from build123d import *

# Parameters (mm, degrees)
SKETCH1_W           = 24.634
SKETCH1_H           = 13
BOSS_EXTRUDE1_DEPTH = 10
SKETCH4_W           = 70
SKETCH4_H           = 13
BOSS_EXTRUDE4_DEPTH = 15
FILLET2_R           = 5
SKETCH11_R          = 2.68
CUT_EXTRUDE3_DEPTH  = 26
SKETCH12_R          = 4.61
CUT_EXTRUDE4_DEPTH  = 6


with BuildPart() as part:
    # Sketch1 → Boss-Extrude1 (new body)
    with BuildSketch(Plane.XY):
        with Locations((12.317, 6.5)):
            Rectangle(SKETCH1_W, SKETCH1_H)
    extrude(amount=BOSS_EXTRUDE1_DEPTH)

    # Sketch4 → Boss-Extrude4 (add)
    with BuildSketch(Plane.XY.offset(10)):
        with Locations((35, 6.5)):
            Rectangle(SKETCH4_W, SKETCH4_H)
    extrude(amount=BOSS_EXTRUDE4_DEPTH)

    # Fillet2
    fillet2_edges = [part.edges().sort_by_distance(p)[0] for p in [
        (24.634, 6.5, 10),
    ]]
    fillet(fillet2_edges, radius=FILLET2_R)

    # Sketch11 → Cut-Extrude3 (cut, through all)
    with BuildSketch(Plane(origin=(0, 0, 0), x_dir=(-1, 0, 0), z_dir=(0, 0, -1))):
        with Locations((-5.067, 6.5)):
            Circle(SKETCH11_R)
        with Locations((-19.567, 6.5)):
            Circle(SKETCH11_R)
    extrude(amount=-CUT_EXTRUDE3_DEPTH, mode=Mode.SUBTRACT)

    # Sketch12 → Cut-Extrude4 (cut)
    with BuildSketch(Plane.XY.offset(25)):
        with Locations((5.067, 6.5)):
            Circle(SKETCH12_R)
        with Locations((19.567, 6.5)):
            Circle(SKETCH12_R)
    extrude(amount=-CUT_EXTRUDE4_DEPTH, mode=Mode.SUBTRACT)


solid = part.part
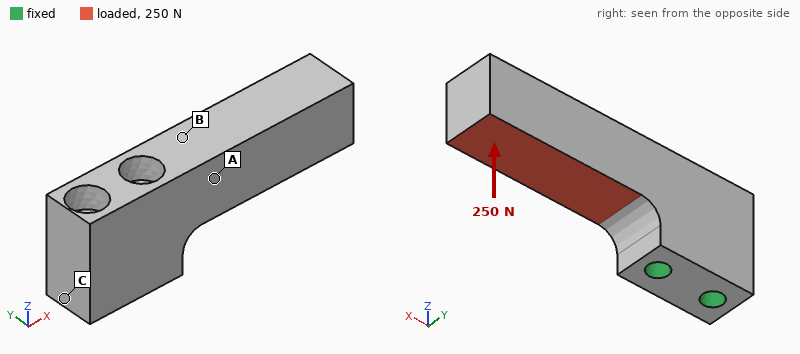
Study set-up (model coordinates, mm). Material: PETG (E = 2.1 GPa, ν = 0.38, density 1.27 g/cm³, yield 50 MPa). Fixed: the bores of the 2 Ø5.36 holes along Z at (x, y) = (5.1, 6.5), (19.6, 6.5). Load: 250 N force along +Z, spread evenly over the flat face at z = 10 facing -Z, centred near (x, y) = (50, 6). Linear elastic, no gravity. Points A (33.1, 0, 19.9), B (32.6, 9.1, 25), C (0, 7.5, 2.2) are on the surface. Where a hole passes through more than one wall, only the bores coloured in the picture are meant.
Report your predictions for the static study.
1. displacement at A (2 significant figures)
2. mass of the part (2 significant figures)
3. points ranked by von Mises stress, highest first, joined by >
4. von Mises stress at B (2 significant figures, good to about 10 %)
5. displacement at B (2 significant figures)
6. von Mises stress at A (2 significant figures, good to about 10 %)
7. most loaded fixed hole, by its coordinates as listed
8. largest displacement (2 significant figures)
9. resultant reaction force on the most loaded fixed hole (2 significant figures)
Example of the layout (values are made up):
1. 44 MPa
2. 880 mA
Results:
1. 0.12 mm
2. 19 g
3. B > A > C
4. 7.8 MPa
5. 0.16 mm
6. 4.2 MPa
7. (19.6, 6.5)
8. 0.81 mm
9. 370 N
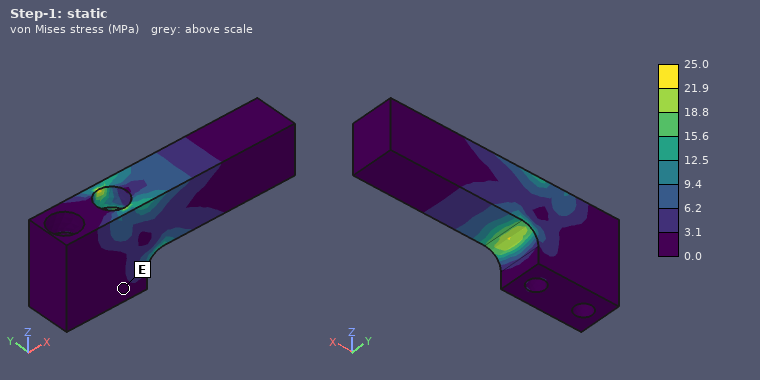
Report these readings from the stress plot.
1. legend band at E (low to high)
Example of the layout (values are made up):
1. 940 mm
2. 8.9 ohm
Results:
1. 0.0 to 3.1 MPa
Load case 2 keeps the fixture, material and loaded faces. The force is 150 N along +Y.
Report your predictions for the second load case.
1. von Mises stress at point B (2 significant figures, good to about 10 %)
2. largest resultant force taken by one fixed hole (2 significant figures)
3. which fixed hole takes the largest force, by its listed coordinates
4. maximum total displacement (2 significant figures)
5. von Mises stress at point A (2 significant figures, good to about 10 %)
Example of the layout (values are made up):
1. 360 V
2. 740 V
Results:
1. 2.3 MPa
2. 270 N
3. (19.6, 6.5)
4. 0.72 mm
5. 6.1 MPa
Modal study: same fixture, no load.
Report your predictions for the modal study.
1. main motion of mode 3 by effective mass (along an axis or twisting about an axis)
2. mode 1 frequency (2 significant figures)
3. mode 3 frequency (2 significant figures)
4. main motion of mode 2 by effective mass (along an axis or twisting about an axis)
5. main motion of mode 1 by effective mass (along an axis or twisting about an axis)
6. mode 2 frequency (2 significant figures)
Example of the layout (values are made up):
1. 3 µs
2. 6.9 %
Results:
1. twisting about X
2. 930 Hz
3. 3400 Hz
4. along Z
5. along Y
6. 1100 Hz
